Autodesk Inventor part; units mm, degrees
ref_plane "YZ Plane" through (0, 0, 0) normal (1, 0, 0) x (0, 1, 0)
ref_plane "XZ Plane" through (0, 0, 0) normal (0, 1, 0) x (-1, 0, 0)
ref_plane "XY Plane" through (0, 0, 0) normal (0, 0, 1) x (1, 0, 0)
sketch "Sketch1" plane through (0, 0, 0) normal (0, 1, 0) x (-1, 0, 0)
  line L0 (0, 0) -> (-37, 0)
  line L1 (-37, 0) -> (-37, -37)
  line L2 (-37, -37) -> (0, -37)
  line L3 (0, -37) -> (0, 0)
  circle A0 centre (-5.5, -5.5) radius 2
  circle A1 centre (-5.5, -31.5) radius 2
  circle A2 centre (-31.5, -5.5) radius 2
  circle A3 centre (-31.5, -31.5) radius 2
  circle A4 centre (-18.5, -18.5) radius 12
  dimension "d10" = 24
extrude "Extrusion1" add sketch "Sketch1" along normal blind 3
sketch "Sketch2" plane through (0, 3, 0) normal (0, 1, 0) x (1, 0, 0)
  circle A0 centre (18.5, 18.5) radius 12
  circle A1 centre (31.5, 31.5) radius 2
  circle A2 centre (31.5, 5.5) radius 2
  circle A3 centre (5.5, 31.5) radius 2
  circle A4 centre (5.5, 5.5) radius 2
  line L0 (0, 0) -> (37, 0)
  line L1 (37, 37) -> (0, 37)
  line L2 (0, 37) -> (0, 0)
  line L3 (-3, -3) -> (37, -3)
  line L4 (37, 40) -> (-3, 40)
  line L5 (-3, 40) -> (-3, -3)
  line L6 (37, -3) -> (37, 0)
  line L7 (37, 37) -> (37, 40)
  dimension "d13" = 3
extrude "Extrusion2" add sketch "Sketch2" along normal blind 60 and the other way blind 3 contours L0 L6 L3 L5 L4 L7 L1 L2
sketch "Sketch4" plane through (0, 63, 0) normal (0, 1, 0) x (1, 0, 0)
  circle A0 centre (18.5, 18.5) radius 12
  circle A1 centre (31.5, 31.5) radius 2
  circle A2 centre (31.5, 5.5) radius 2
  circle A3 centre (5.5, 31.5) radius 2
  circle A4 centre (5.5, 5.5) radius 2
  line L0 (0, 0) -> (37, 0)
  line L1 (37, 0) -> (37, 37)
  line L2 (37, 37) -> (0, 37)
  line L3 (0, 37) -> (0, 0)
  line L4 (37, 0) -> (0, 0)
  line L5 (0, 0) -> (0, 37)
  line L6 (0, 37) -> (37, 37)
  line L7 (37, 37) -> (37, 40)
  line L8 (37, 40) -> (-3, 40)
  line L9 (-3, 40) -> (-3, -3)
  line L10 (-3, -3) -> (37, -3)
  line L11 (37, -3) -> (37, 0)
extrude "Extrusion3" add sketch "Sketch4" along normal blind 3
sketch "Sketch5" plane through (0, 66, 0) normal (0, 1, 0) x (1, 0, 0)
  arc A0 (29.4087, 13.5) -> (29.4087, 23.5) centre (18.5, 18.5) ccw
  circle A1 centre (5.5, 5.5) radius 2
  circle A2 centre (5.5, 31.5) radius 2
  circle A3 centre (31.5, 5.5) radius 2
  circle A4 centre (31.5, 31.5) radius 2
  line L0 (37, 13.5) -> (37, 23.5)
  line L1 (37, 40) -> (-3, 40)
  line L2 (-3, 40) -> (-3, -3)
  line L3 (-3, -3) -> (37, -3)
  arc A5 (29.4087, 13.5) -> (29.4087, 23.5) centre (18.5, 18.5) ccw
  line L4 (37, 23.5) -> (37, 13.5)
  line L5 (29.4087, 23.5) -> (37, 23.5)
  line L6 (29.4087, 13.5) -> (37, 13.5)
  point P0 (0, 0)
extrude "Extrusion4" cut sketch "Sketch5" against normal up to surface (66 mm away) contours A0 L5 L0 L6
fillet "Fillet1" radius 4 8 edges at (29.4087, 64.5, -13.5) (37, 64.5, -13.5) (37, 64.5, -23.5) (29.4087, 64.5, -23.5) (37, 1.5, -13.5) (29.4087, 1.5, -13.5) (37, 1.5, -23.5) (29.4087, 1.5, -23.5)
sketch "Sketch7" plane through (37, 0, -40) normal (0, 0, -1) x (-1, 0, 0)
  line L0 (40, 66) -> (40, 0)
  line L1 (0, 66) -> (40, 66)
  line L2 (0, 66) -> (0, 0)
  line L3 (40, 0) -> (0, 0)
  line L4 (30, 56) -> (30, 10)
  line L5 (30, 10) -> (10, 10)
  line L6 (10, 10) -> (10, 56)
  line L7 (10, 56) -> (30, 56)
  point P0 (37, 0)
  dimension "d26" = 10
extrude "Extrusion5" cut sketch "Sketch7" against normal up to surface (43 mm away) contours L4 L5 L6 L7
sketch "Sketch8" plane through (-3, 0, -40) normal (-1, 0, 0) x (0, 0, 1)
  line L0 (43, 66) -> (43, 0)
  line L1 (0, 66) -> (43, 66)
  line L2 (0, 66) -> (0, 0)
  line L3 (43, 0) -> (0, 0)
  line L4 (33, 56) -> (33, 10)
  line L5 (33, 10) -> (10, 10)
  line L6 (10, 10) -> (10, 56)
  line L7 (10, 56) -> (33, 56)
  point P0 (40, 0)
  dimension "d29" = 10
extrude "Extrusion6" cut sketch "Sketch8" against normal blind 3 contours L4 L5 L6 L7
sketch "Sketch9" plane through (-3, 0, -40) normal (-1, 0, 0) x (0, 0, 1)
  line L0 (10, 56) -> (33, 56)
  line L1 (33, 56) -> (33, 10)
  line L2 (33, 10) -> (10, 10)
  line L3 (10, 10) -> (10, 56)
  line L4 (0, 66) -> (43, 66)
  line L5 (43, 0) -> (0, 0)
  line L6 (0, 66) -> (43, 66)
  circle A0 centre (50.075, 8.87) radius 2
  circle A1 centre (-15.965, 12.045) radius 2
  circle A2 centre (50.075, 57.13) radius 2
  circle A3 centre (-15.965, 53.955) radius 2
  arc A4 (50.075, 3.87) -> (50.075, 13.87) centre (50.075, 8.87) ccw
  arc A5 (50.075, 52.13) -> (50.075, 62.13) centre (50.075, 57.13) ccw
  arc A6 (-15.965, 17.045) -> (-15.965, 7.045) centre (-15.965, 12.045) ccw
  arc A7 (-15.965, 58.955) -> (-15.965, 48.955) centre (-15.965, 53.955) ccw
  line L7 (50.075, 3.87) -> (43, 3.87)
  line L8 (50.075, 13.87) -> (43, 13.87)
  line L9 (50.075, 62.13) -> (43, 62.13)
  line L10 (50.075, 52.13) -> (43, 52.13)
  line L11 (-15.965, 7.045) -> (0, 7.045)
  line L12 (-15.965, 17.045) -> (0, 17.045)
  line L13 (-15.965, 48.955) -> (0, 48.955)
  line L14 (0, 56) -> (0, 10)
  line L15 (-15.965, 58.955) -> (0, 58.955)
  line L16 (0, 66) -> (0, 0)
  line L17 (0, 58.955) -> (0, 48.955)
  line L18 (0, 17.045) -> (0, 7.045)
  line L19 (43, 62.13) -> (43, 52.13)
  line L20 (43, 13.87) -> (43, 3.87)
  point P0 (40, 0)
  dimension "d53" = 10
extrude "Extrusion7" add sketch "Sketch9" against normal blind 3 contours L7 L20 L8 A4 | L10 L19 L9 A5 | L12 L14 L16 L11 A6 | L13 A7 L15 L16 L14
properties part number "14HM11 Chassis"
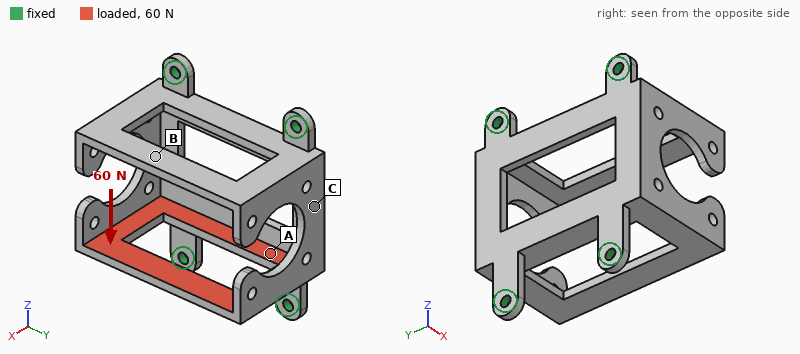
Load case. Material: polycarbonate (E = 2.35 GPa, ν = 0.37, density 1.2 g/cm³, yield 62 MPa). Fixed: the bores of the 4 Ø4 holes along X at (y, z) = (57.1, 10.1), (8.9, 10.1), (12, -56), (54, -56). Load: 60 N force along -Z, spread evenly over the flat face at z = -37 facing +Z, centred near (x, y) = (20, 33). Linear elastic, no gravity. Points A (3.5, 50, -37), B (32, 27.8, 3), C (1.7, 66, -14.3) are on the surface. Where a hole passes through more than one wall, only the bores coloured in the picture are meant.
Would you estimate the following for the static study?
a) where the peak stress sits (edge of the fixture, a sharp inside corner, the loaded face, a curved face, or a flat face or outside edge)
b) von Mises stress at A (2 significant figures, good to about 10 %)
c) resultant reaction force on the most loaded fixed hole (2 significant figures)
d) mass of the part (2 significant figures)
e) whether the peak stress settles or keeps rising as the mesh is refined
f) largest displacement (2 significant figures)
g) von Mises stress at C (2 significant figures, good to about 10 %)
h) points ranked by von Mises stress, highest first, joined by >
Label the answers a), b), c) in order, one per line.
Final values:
a) edge of the fixture
b) 1.3 MPa
c) 22 N
d) 25 g
e) keeps rising
f) 1.0 mm
g) 2.2 MPa
h) C > A > B
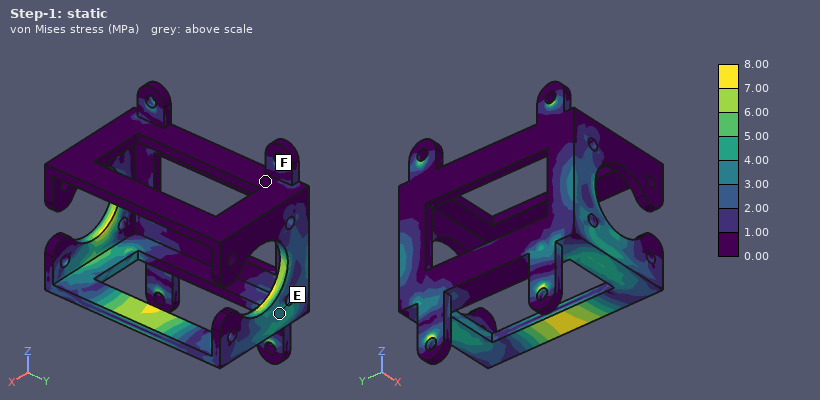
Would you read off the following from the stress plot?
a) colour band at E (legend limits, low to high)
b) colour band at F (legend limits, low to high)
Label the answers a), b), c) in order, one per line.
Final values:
a) 3.00 to 4.00 MPa
b) 0.00 to 1.00 MPa
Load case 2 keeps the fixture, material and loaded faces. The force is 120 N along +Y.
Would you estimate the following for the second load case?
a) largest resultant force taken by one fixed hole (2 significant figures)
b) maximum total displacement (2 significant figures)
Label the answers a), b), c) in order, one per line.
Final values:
a) 59 N
b) 1.3 mm
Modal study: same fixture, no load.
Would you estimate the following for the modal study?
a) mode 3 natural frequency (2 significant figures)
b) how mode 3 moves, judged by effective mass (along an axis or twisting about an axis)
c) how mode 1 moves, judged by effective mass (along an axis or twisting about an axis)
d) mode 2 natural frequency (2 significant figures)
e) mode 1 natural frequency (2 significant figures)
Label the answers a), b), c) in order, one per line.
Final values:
a) 650 Hz
b) along Z
c) along Y
d) 570 Hz
e) 520 Hz
